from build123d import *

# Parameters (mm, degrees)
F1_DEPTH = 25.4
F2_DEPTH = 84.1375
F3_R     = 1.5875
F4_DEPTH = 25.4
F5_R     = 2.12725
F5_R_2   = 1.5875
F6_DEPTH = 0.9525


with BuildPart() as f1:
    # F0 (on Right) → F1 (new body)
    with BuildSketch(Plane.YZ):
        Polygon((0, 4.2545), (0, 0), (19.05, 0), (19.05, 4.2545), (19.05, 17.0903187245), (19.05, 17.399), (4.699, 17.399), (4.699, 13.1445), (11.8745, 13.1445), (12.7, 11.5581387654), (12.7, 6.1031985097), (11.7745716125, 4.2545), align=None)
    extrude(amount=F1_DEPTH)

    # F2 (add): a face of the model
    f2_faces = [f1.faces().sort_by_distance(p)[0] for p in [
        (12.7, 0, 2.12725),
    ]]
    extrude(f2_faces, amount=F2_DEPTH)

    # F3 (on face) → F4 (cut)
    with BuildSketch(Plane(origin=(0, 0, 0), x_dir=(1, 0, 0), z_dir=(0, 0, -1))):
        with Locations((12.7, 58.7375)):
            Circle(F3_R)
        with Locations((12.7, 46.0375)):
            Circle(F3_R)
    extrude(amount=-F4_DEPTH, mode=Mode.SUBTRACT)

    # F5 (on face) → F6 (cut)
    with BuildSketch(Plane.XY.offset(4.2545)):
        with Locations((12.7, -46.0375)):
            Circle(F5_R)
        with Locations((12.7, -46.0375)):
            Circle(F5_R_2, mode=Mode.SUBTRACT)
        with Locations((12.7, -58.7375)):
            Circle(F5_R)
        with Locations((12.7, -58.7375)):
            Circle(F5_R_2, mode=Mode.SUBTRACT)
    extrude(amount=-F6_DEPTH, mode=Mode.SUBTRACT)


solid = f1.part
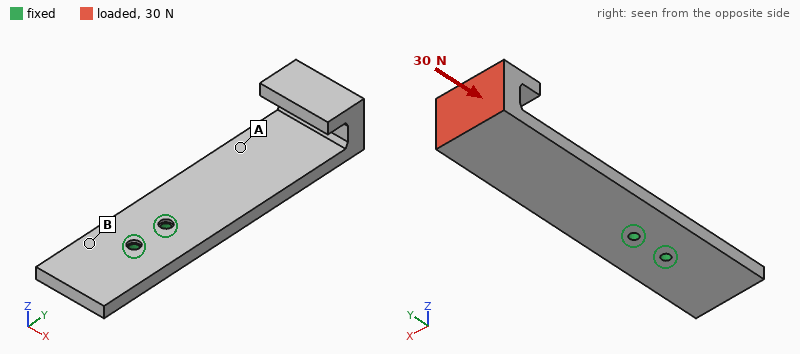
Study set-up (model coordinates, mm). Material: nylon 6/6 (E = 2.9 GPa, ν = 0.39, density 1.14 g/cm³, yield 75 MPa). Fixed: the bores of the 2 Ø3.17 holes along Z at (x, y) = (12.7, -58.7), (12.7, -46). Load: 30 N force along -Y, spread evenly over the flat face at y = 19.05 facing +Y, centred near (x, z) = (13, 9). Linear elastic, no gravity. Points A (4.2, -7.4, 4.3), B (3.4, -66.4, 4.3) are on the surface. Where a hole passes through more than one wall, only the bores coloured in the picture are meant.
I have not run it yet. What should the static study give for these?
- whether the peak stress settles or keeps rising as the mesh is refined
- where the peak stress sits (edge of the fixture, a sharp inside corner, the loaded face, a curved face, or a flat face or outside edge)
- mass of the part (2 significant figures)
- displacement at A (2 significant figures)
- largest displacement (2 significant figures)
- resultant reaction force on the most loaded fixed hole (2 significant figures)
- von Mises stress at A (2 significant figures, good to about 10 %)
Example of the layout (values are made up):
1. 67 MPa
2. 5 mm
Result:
1. keeps rising
2. edge of the fixture
3. 16 g
4. 0.34 mm
5. 0.99 mm
6. 18 N
7. 2.8 MPa
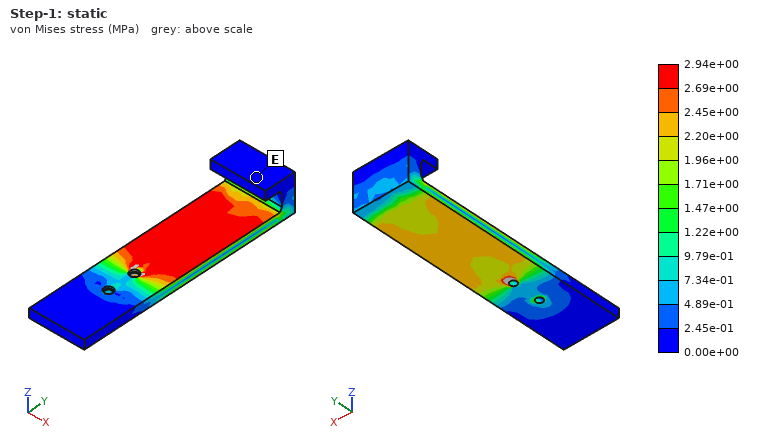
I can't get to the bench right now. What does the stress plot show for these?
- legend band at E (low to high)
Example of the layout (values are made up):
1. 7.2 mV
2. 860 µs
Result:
1. 0.00e+00 to 2.45e-01 MPa
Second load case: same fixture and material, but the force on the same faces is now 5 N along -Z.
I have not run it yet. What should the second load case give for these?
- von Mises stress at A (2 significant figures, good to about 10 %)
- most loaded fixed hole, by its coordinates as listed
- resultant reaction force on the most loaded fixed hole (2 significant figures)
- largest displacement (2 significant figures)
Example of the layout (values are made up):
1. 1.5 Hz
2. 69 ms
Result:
1. 1.7 MPa
2. (12.7, -46)
3. 20 N
4. 1.1 mm
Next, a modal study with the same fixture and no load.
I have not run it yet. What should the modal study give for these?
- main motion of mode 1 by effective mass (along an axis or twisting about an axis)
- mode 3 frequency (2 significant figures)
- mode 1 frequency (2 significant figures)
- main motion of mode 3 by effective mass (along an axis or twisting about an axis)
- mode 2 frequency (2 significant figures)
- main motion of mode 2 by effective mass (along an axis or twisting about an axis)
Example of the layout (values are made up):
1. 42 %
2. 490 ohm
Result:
1. along Z
2. 870 Hz
3. 160 Hz
4. along X
5. 510 Hz
6. along X
